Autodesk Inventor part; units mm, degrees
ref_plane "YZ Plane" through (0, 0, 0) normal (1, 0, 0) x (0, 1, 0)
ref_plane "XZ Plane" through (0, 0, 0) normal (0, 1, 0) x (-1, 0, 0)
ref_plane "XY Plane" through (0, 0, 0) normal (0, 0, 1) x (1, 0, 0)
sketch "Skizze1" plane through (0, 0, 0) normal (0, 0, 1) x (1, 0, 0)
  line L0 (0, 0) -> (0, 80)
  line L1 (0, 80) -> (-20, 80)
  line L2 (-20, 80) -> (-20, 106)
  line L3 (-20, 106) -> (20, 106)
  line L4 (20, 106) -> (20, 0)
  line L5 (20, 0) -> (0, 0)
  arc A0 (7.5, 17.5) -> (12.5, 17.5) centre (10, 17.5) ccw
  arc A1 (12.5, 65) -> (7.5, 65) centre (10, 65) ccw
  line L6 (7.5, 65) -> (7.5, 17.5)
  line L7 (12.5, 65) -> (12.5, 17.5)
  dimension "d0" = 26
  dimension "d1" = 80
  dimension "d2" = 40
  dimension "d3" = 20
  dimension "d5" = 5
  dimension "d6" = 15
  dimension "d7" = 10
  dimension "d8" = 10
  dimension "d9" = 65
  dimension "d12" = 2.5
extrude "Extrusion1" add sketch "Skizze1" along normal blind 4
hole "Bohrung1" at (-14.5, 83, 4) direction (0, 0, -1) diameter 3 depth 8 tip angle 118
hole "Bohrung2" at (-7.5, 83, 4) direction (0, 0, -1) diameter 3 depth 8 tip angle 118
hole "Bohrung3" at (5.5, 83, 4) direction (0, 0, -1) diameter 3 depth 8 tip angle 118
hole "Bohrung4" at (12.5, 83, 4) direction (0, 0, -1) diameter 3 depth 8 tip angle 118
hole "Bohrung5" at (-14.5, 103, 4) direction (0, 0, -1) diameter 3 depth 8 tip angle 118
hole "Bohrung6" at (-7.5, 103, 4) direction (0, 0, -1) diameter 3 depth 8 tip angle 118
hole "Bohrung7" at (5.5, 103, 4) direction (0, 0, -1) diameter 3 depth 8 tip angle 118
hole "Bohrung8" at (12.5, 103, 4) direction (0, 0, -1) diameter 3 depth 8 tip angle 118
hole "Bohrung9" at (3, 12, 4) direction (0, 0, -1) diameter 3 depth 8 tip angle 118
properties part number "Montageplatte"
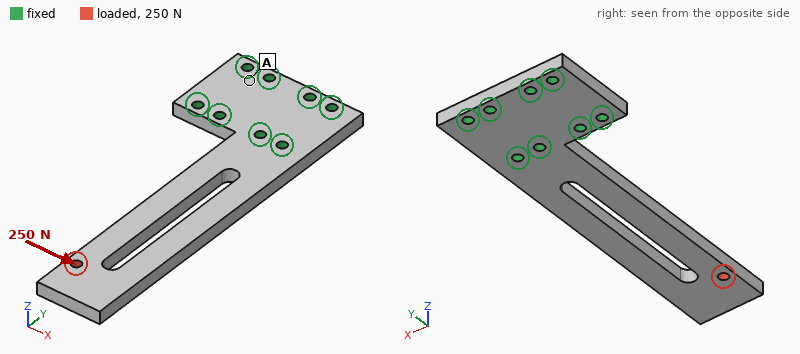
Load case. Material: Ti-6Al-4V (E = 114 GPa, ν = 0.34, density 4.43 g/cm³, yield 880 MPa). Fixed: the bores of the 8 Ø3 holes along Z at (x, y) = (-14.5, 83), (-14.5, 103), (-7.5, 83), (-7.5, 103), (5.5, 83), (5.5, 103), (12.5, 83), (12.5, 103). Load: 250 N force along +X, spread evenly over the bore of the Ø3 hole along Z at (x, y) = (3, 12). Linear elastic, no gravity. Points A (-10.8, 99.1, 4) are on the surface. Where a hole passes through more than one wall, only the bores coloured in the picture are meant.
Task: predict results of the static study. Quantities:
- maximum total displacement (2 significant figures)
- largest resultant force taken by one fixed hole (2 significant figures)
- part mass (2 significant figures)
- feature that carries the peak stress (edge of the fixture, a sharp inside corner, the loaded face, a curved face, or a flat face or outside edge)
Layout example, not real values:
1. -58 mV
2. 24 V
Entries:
1. 0.25 mm
2. 1.2 kN
3. 41 g
4. a curved face
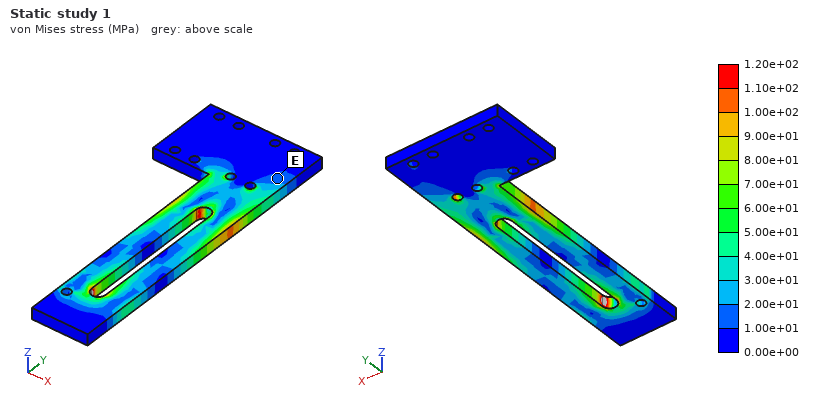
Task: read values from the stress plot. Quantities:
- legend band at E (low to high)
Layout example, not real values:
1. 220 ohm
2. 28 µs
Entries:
1. 1.00e+01 to 2.00e+01 MPa
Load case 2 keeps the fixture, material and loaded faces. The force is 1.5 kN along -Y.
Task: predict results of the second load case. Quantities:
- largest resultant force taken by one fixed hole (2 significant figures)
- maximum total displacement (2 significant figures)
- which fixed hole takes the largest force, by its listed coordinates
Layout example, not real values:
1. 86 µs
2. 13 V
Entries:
1. 1.2 kN
2. 0.13 mm
3. (5.5, 83)
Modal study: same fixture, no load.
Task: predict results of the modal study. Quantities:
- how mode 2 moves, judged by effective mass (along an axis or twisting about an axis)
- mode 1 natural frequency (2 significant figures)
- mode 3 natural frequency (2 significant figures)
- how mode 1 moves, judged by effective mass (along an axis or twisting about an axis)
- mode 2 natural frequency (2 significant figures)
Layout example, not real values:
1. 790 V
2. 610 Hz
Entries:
1. along X
2. 480 Hz
3. 2900 Hz
4. along Z
5. 1700 Hz
